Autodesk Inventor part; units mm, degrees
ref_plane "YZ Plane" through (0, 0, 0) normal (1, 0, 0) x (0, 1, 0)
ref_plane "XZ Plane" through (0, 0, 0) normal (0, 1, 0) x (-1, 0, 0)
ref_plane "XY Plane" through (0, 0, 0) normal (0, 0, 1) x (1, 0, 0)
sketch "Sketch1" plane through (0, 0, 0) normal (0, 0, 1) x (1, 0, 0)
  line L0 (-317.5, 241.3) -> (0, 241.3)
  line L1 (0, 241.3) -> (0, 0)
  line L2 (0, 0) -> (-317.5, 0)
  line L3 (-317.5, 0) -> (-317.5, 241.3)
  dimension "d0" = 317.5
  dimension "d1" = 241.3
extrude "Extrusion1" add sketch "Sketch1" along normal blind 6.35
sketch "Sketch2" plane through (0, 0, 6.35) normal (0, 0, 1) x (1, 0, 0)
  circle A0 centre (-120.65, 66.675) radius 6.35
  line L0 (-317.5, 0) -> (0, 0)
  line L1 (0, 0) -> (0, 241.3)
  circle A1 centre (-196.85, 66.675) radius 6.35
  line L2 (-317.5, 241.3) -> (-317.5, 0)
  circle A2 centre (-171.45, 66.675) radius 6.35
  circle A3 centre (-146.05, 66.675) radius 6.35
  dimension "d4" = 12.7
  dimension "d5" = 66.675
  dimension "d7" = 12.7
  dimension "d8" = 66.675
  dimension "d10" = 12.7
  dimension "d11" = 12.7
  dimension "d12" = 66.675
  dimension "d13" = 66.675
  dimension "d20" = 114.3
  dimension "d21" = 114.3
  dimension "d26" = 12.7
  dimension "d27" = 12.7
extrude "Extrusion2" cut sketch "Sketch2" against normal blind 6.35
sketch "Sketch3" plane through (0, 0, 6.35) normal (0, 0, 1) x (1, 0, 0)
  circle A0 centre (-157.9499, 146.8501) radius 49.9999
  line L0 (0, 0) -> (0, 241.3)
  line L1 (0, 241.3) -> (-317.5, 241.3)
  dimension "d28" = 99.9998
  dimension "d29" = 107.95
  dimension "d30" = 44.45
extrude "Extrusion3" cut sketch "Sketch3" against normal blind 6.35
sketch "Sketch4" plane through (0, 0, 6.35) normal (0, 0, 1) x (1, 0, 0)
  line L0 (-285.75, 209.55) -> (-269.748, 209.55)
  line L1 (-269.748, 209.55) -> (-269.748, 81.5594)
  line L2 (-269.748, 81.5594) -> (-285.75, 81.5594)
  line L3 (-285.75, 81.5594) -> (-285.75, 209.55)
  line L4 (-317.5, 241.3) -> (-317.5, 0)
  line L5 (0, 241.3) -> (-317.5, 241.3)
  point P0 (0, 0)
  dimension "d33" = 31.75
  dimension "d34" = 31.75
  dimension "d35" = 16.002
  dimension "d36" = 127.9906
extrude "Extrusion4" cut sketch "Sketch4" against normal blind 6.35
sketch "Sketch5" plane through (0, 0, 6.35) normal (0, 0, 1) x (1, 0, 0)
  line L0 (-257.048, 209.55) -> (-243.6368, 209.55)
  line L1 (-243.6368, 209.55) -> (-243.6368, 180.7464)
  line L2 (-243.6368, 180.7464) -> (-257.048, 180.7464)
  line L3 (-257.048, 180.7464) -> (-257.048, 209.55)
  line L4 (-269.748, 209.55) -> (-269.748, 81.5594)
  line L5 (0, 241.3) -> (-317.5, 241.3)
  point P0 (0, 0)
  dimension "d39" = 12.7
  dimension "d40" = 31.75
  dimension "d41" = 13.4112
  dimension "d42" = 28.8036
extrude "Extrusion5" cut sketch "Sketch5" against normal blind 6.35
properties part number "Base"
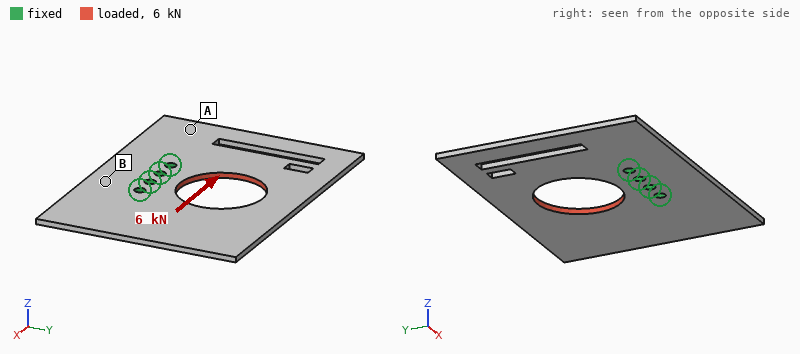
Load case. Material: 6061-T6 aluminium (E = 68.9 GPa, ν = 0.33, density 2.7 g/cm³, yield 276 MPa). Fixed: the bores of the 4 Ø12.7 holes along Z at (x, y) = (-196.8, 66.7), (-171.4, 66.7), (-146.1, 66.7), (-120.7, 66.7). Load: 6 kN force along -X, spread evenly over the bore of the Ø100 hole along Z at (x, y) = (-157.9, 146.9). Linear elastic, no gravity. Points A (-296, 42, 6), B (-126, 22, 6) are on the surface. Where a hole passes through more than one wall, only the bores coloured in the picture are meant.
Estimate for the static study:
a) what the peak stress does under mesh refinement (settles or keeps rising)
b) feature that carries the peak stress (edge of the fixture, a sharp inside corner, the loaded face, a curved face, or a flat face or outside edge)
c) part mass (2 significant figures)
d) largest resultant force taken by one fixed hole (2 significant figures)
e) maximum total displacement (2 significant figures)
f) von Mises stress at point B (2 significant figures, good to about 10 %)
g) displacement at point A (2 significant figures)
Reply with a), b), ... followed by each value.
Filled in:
a) keeps rising
b) edge of the fixture
c) 1.1 kg
d) 5.5 kN
e) 0.14 mm
f) 8.4 MPa
g) 0.058 mm
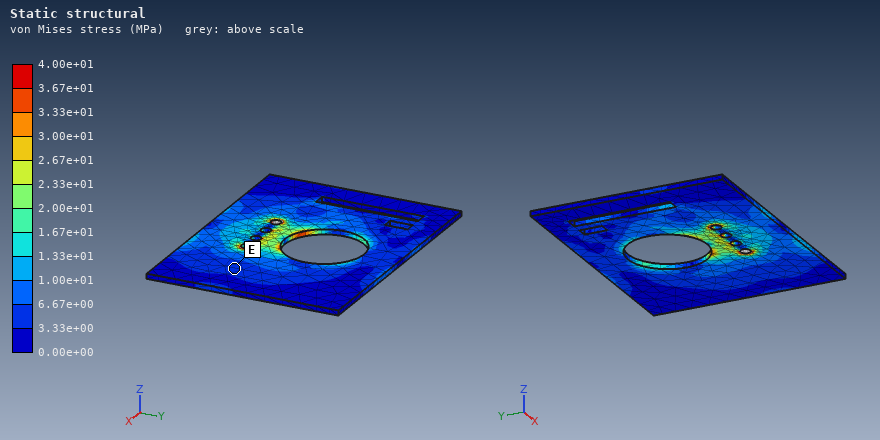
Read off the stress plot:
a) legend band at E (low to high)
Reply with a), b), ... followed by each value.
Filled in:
a) 3.33e+00 to 6.67e+00 MPa
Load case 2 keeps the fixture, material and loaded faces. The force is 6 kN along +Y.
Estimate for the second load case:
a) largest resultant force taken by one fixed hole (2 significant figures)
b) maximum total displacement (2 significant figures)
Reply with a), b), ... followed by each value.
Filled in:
a) 2.6 kN
b) 26 µm
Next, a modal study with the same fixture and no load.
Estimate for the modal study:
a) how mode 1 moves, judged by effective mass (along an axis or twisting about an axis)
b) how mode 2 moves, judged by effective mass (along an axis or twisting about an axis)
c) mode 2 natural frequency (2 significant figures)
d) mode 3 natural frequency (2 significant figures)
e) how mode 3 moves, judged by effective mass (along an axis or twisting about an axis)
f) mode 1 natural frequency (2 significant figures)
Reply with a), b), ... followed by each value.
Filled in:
a) along Z
b) twisting about Y
c) 170 Hz
d) 310 Hz
e) along Z
f) 130 Hz
